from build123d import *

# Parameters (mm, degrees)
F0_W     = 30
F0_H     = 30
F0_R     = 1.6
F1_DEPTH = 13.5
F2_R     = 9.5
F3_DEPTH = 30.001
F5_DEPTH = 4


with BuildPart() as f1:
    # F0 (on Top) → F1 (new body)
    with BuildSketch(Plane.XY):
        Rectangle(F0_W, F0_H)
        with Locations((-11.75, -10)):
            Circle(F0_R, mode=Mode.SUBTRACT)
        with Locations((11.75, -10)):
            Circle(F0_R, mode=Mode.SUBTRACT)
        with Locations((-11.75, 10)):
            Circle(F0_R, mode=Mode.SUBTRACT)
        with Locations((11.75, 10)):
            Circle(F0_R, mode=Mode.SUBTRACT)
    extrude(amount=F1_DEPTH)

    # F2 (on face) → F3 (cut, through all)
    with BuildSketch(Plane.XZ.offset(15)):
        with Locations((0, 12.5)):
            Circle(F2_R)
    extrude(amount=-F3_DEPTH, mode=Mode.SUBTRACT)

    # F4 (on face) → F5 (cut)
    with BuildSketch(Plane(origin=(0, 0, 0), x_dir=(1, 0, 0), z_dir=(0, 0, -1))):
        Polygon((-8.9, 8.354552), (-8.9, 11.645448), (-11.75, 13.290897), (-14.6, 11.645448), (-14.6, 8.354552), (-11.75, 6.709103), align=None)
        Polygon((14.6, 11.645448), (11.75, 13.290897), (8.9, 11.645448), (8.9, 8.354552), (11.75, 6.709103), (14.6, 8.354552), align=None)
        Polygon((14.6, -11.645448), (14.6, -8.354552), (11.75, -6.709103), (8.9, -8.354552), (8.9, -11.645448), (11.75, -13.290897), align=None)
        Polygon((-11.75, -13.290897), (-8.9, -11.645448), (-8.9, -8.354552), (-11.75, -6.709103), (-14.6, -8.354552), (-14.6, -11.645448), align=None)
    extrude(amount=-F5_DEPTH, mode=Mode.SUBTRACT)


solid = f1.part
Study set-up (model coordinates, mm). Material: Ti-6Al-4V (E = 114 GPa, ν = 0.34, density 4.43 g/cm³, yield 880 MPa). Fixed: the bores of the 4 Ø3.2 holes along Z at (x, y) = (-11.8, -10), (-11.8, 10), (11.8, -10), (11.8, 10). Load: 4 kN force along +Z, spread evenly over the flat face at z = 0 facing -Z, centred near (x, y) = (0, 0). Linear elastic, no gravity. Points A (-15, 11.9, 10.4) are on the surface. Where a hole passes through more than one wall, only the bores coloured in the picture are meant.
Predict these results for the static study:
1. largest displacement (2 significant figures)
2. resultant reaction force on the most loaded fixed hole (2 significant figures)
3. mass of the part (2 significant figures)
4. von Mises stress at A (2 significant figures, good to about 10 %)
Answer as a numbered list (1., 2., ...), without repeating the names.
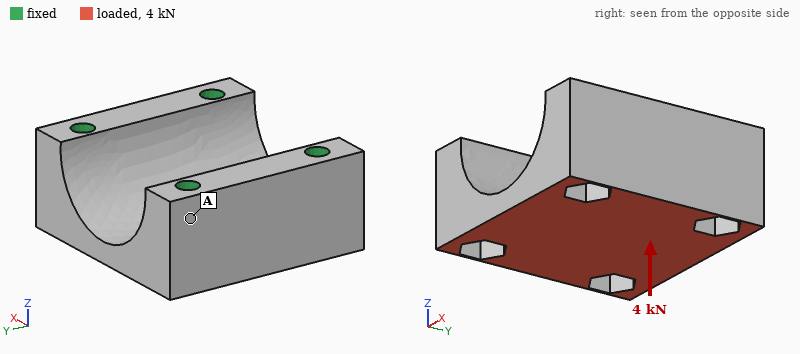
1. 4.2 µm
2. 1.2 kN
3. 29 g
4. 6.2 MPa
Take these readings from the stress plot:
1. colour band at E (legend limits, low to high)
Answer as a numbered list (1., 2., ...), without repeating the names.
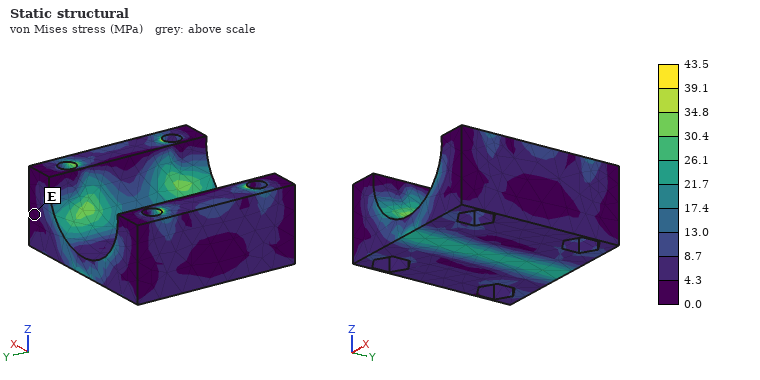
1. 0.0 to 4.3 MPa
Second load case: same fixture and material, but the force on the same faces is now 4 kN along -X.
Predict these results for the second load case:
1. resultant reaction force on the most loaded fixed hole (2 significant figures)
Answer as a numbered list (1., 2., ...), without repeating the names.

1. 1.1 kN
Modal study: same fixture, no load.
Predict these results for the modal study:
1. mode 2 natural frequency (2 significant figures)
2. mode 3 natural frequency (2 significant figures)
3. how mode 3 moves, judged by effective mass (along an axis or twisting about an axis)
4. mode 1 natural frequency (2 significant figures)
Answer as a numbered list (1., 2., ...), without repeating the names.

1. 47 kHz
2. 53 kHz
3. along Y
4. 46 kHz
